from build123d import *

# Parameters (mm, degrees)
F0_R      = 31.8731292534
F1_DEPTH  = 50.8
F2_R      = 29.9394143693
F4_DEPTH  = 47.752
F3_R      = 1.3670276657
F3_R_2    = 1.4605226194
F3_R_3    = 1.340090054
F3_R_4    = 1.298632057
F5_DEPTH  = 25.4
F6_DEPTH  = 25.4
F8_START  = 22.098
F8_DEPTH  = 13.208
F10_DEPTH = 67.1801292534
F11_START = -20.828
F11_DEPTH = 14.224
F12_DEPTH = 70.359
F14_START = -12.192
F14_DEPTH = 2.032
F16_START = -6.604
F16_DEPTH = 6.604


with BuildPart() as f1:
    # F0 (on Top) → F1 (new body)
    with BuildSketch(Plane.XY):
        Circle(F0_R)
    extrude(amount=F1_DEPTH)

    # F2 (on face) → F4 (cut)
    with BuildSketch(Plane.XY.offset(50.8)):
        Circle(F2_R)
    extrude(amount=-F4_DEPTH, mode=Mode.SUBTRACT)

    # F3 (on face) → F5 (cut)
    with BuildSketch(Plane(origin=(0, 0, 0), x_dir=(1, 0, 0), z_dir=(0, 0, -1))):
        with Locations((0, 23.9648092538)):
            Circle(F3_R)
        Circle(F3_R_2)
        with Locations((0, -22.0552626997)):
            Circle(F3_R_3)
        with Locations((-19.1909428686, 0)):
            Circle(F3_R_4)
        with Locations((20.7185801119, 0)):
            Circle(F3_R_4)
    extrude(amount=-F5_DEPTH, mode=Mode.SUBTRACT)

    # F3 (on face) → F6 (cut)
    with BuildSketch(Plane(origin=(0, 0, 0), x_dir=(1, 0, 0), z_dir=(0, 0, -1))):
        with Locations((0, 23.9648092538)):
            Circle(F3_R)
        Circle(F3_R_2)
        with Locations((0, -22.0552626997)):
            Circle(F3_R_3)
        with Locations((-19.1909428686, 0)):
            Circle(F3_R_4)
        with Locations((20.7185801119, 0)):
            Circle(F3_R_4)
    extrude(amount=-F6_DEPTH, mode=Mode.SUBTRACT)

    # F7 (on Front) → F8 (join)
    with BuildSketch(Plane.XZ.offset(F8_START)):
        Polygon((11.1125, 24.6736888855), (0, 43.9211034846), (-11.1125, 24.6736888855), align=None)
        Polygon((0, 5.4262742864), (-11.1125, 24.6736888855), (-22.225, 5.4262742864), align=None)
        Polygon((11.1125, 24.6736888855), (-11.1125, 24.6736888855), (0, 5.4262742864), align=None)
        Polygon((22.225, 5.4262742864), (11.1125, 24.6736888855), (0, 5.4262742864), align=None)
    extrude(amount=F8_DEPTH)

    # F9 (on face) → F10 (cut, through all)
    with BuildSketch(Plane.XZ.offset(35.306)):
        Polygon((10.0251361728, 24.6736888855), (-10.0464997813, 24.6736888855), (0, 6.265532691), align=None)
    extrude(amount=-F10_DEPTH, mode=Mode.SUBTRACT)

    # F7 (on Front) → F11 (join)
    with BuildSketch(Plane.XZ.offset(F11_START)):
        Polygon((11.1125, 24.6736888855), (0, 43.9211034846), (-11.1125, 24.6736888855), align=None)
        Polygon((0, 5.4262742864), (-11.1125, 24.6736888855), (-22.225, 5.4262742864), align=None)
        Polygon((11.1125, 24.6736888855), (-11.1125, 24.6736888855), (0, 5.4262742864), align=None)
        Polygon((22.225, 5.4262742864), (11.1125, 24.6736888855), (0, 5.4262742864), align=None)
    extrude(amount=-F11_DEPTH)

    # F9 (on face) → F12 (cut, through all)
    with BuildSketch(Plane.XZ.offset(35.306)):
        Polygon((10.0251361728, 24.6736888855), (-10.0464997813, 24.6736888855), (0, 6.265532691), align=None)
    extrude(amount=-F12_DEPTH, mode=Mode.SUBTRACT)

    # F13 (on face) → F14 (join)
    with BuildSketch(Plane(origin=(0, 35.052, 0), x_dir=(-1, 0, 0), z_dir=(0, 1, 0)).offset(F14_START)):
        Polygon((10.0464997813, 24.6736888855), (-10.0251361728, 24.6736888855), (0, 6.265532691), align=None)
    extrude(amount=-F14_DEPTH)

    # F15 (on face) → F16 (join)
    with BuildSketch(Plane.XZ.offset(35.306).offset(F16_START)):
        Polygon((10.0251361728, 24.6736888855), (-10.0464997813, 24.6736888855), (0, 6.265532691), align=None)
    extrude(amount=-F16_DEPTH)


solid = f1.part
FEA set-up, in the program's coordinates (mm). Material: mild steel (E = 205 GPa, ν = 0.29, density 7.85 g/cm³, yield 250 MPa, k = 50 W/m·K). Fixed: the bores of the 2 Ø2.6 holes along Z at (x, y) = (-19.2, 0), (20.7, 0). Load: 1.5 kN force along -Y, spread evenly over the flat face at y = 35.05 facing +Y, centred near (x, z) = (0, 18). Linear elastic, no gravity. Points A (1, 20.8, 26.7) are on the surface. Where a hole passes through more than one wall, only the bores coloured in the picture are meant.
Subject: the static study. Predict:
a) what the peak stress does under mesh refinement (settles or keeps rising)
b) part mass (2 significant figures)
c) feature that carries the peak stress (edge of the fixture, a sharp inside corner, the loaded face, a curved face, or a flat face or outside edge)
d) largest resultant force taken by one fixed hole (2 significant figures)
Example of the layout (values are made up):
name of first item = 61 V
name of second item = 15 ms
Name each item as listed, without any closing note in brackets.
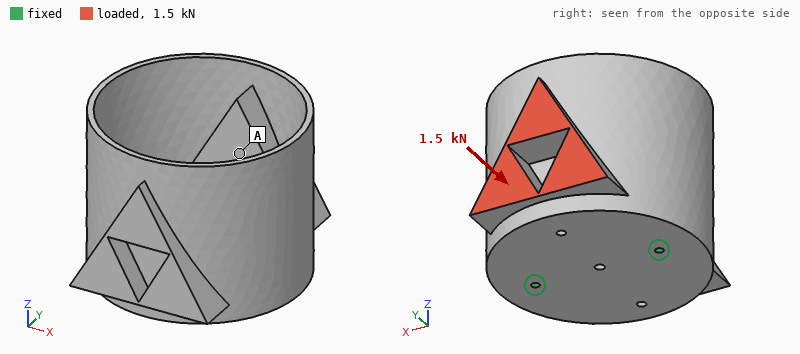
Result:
what the peak stress does under mesh refinement = keeps rising
part mass = 350 g
feature that carries the peak stress = edge of the fixture
largest resultant force taken by one fixed hole = 790 N
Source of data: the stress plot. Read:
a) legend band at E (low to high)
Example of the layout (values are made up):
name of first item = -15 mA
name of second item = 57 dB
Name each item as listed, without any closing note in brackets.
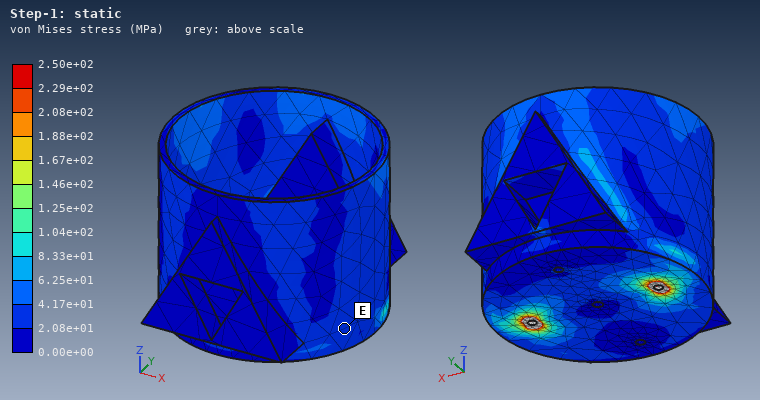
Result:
legend band at E = 2.08e+01 to 4.17e+01 MPa
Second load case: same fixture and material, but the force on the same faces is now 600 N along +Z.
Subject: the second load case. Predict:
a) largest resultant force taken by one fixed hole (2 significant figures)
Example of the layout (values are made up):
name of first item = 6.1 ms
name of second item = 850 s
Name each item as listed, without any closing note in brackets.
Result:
largest resultant force taken by one fixed hole = 310 N
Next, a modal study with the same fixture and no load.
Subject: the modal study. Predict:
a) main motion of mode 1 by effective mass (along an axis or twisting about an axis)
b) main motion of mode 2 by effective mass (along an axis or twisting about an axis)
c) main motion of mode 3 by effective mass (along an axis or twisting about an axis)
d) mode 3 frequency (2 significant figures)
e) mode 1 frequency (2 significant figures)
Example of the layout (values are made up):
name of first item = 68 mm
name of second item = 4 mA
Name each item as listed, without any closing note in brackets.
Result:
main motion of mode 1 by effective mass = along Y
main motion of mode 2 by effective mass = along Z
main motion of mode 3 by effective mass = along X
mode 3 frequency = 2200 Hz
mode 1 frequency = 600 Hz
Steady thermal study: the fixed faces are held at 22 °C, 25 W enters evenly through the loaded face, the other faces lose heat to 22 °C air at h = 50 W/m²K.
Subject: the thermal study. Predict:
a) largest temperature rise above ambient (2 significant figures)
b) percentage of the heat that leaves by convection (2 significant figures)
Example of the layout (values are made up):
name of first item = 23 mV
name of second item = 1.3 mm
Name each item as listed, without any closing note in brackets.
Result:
largest temperature rise above ambient = 41 K
percentage of the heat that leaves by convection = 75 %
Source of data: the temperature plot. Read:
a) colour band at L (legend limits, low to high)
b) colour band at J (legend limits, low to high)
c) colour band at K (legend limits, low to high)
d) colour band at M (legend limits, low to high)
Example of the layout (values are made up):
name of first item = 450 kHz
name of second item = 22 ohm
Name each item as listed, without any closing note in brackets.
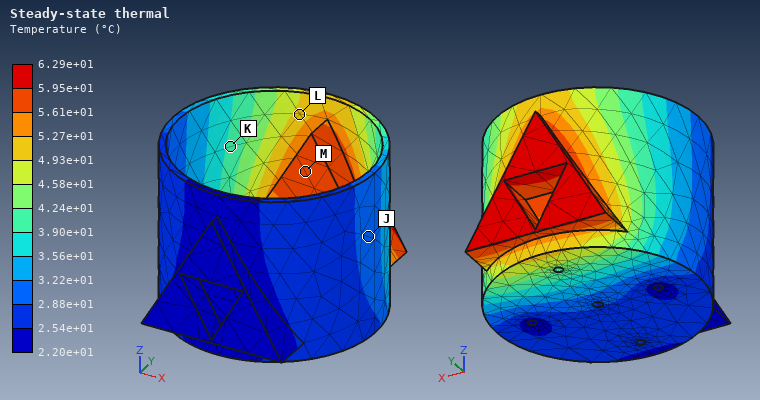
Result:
colour band at L = 4.93e+01 to 5.27e+01 °C
colour band at J = 2.88e+01 to 3.22e+01 °C
colour band at K = 3.90e+01 to 4.24e+01 °C
colour band at M = 5.61e+01 to 5.95e+01 °C
